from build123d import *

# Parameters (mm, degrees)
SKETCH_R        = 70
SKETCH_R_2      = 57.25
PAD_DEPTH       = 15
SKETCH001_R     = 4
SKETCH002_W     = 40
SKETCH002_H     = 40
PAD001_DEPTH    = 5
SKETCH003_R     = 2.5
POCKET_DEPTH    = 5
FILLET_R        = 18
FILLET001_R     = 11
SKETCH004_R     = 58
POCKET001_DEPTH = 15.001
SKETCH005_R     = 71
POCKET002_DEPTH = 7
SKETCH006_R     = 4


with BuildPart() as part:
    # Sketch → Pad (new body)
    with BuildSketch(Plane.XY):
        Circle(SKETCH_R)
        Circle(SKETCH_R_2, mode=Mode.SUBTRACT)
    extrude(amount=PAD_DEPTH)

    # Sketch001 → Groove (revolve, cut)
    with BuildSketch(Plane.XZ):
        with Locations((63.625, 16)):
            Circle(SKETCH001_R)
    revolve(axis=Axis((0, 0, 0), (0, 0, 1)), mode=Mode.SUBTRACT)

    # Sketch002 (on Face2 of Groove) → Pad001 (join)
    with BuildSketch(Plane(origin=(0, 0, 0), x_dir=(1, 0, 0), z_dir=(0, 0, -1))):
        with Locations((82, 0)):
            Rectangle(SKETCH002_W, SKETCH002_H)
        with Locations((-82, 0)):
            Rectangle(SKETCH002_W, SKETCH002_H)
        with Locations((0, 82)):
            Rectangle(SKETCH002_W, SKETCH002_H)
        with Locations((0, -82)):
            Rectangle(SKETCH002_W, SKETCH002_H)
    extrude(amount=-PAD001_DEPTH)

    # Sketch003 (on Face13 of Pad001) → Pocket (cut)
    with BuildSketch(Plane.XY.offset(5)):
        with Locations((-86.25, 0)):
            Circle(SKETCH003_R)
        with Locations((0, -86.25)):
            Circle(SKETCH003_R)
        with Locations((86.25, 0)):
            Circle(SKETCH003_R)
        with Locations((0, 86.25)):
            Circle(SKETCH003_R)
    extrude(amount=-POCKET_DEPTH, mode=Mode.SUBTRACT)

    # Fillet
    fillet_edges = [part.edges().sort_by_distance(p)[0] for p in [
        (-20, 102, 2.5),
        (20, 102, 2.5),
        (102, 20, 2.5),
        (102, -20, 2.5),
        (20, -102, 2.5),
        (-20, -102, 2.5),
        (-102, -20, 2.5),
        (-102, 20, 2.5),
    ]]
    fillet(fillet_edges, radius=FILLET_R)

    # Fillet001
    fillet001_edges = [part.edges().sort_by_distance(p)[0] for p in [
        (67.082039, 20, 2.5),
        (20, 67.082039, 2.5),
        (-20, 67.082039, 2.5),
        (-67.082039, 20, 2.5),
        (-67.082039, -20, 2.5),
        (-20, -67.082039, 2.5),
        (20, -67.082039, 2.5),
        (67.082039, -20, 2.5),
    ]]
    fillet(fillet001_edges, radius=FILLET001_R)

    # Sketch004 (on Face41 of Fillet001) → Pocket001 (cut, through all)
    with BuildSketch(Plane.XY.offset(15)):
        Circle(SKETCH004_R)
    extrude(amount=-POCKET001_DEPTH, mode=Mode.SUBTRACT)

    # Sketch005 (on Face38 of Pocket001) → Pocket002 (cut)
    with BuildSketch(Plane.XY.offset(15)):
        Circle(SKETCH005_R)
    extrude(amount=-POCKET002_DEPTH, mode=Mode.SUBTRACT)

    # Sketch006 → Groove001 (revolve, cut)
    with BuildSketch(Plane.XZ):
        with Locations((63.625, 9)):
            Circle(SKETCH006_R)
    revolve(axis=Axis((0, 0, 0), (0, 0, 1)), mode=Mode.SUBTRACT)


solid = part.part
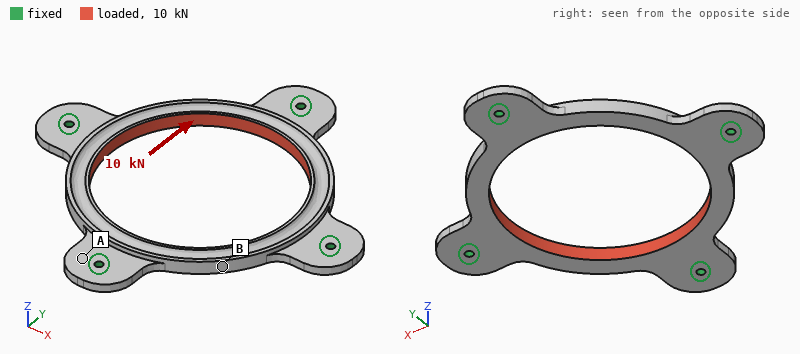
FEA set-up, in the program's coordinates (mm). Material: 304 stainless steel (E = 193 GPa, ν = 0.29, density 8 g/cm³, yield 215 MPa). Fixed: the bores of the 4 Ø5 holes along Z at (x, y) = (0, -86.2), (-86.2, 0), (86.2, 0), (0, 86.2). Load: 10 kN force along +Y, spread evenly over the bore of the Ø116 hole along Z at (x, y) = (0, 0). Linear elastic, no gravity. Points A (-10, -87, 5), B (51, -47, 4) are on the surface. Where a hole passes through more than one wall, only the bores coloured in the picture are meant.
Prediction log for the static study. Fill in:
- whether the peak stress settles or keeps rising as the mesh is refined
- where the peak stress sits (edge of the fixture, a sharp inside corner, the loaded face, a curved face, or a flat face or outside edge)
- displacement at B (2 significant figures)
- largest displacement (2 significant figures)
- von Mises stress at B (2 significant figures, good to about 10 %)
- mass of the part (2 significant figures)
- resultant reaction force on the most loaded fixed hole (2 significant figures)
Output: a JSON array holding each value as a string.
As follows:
["keeps rising", "edge of the fixture", "33 µm", "37 µm", "38 MPa", "440 g", "2.6 kN"]
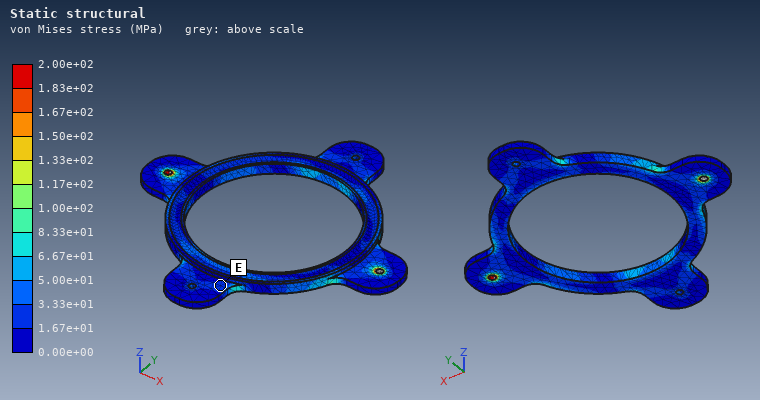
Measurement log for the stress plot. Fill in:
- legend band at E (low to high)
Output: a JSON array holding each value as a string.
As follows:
["1.67e+01 to 3.33e+01 MPa"]
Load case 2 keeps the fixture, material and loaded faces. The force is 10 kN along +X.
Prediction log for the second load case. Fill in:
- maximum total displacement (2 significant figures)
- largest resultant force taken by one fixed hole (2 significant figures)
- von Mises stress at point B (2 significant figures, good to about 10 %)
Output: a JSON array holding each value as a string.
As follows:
["37 µm", "2.6 kN", "31 MPa"]
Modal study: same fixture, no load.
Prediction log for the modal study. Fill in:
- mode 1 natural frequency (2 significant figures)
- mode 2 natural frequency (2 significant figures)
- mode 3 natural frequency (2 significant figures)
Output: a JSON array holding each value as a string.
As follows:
["2200 Hz", "2300 Hz", "2300 Hz"]
